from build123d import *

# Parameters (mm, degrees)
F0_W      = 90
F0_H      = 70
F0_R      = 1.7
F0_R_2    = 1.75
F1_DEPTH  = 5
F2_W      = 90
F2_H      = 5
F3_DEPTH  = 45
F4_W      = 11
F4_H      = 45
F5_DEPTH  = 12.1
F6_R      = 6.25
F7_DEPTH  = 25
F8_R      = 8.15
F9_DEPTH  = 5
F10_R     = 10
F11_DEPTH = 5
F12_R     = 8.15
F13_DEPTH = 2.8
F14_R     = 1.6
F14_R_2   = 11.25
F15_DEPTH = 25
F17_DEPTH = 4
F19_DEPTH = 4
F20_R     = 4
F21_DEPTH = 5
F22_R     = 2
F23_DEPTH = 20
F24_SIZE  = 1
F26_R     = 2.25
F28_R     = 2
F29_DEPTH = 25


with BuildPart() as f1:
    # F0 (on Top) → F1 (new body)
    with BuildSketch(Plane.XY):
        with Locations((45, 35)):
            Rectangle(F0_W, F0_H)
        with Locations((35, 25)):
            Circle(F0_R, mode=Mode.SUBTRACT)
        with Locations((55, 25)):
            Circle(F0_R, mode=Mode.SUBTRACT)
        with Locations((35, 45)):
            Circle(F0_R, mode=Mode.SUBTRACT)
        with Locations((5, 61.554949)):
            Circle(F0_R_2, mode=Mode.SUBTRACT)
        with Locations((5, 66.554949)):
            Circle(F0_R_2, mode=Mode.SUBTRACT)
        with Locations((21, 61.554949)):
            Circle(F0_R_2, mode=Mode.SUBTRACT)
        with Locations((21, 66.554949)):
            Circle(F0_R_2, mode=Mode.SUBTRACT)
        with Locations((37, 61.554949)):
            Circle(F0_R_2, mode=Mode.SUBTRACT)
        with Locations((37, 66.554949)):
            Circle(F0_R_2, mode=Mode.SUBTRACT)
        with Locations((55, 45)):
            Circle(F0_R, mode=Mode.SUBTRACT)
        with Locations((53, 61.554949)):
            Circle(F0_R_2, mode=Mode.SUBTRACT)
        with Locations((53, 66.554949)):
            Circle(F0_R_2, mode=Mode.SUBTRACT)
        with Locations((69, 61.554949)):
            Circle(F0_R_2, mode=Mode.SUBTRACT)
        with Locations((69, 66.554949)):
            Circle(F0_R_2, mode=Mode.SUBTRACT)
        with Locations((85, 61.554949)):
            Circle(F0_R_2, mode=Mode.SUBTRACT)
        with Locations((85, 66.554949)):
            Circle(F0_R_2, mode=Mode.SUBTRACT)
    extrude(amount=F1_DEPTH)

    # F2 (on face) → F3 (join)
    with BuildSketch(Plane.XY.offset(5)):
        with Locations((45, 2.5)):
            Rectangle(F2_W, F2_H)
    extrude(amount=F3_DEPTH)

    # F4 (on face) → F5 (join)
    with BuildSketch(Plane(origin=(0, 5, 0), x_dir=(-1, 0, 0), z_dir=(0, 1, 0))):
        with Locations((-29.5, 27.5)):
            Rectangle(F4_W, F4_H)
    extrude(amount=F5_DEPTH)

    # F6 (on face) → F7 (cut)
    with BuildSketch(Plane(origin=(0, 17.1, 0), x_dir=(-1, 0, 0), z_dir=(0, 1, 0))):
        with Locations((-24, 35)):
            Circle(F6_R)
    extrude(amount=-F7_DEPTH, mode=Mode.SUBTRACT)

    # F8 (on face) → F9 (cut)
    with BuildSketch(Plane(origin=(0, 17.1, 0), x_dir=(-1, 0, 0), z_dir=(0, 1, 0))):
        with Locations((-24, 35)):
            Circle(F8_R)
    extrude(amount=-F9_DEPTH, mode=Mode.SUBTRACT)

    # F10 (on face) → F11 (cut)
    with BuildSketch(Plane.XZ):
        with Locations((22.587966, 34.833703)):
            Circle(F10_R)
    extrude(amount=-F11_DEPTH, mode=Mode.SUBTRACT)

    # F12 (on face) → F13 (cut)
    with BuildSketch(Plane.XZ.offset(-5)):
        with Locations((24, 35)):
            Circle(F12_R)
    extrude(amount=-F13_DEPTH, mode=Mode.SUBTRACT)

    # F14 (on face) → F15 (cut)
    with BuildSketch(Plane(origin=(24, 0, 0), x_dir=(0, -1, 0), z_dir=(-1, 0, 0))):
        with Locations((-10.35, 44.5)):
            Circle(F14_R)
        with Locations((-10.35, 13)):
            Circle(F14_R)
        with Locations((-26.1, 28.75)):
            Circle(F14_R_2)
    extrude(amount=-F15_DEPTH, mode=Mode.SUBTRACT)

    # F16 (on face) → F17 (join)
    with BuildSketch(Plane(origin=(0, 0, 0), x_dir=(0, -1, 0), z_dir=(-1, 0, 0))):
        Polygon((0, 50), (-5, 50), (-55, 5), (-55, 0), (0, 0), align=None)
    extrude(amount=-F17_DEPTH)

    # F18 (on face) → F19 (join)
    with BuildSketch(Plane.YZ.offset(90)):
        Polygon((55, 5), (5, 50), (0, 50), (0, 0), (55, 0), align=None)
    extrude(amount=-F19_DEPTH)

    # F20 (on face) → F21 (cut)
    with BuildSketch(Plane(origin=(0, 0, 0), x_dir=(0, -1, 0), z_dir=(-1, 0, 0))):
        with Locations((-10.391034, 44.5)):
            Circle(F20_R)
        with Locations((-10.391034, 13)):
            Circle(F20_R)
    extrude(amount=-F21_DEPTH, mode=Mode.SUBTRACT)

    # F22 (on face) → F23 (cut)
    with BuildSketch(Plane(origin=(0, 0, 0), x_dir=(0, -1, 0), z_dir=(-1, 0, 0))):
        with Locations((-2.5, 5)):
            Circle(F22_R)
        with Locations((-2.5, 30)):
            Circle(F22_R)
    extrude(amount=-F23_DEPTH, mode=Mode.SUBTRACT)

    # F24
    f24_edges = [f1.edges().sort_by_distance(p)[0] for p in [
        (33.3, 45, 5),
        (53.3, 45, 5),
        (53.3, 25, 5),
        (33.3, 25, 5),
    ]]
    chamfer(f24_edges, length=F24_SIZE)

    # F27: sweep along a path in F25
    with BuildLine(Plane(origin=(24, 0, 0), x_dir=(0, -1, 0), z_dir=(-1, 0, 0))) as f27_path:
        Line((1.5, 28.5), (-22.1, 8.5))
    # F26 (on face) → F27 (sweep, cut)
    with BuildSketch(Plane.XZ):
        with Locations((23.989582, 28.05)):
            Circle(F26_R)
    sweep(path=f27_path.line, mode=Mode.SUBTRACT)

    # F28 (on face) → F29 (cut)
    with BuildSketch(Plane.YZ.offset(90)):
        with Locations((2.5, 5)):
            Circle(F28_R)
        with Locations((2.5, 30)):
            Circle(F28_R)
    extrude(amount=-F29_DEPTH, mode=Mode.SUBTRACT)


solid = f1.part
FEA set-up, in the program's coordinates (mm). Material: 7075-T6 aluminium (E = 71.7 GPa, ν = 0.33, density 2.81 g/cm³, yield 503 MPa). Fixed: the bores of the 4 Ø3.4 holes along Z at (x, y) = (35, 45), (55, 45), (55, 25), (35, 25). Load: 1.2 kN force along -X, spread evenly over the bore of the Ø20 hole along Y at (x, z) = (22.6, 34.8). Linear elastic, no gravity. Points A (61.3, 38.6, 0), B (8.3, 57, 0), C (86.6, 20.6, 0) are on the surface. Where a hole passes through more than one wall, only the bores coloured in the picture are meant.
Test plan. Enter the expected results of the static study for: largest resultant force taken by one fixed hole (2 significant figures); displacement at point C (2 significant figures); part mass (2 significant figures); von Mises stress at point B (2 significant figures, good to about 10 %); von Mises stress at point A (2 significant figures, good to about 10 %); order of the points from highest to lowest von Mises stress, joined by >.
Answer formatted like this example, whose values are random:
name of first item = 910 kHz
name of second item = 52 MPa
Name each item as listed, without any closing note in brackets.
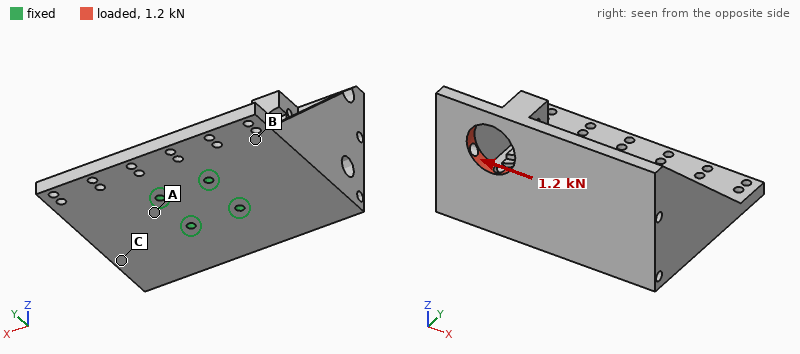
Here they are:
largest resultant force taken by one fixed hole = 1.6 kN
displacement at point C = 0.12 mm
part mass = 170 g
von Mises stress at point B = 16 MPa
von Mises stress at point A = 35 MPa
order of the points from highest to lowest von Mises stress, joined by > = A > B > C
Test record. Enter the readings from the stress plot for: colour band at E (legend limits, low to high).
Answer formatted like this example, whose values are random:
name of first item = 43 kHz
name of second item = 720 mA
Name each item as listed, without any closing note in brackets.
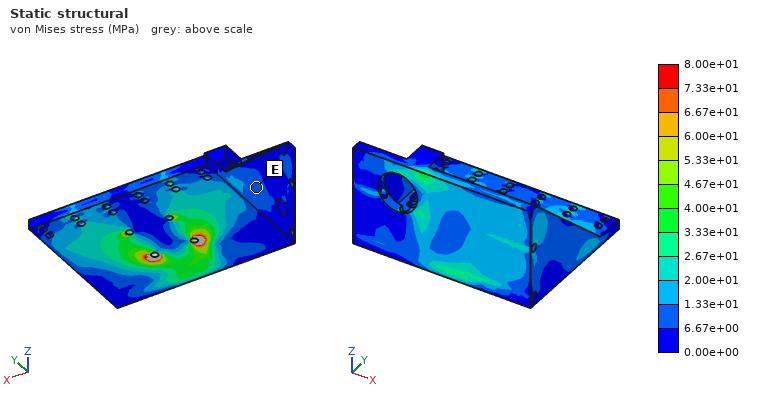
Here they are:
colour band at E = 6.67e+00 to 1.33e+01 MPa
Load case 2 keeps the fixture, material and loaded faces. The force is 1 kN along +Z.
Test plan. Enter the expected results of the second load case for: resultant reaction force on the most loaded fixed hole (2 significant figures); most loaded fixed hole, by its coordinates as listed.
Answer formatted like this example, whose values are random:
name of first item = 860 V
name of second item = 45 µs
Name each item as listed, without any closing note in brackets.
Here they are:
resultant reaction force on the most loaded fixed hole = 1.6 kN
most loaded fixed hole, by its coordinates as listed = (35, 25)
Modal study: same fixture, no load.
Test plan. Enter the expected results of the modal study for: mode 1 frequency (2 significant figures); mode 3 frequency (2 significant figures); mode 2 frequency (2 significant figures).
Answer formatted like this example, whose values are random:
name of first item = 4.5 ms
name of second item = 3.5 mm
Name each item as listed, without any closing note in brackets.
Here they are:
mode 1 frequency = 1300 Hz
mode 3 frequency = 2600 Hz
mode 2 frequency = 1400 Hz
